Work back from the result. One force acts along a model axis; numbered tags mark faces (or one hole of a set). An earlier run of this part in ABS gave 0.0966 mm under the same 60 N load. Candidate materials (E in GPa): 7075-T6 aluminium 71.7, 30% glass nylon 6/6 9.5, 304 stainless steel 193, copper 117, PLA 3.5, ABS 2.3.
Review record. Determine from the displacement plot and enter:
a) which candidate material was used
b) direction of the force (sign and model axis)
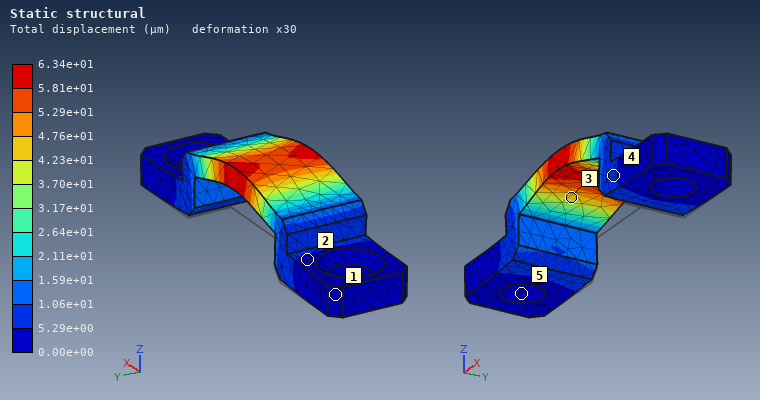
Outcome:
PLA
+Z
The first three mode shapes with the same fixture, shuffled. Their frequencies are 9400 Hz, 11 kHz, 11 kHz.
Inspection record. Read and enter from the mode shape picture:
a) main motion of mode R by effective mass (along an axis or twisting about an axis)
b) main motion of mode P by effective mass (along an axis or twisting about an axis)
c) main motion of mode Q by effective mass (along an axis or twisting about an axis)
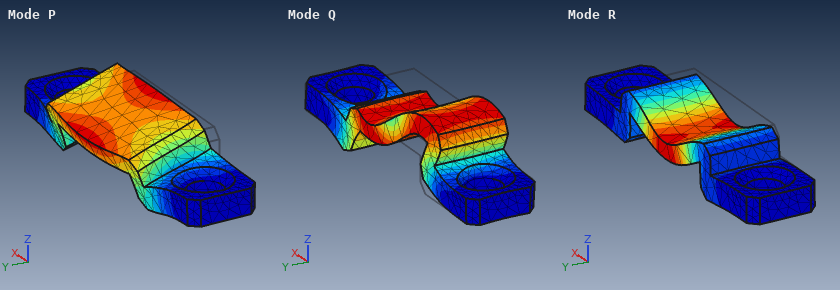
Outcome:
along Z
along Y
along X
